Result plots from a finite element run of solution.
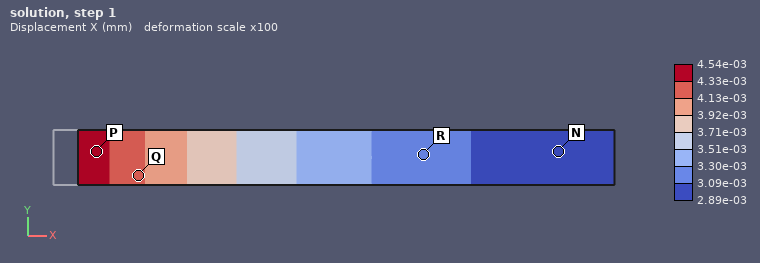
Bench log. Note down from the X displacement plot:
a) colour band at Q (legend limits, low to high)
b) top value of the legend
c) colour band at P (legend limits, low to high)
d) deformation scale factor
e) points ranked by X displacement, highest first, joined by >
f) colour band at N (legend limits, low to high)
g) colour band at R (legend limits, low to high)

4.13e-03 to 4.33e-03 mm
4.54e-03 mm
4.33e-03 to 4.54e-03 mm
100
P > Q > R > N
2.89e-03 to 3.09e-03 mm
3.09e-03 to 3.30e-03 mm
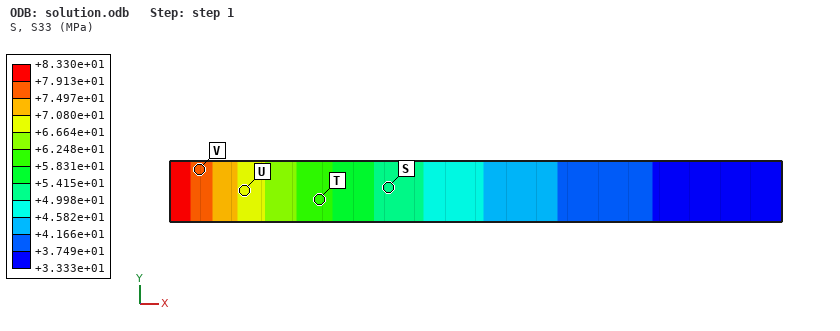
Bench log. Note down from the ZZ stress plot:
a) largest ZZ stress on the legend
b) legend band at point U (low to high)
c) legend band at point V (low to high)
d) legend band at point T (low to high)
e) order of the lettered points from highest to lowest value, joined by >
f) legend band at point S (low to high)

+8.330e+01 MPa
+6.664e+01 to +7.080e+01 MPa
+7.497e+01 to +7.913e+01 MPa
+5.831e+01 to +6.248e+01 MPa
V > U > T > S
+4.998e+01 to +5.415e+01 MPa
